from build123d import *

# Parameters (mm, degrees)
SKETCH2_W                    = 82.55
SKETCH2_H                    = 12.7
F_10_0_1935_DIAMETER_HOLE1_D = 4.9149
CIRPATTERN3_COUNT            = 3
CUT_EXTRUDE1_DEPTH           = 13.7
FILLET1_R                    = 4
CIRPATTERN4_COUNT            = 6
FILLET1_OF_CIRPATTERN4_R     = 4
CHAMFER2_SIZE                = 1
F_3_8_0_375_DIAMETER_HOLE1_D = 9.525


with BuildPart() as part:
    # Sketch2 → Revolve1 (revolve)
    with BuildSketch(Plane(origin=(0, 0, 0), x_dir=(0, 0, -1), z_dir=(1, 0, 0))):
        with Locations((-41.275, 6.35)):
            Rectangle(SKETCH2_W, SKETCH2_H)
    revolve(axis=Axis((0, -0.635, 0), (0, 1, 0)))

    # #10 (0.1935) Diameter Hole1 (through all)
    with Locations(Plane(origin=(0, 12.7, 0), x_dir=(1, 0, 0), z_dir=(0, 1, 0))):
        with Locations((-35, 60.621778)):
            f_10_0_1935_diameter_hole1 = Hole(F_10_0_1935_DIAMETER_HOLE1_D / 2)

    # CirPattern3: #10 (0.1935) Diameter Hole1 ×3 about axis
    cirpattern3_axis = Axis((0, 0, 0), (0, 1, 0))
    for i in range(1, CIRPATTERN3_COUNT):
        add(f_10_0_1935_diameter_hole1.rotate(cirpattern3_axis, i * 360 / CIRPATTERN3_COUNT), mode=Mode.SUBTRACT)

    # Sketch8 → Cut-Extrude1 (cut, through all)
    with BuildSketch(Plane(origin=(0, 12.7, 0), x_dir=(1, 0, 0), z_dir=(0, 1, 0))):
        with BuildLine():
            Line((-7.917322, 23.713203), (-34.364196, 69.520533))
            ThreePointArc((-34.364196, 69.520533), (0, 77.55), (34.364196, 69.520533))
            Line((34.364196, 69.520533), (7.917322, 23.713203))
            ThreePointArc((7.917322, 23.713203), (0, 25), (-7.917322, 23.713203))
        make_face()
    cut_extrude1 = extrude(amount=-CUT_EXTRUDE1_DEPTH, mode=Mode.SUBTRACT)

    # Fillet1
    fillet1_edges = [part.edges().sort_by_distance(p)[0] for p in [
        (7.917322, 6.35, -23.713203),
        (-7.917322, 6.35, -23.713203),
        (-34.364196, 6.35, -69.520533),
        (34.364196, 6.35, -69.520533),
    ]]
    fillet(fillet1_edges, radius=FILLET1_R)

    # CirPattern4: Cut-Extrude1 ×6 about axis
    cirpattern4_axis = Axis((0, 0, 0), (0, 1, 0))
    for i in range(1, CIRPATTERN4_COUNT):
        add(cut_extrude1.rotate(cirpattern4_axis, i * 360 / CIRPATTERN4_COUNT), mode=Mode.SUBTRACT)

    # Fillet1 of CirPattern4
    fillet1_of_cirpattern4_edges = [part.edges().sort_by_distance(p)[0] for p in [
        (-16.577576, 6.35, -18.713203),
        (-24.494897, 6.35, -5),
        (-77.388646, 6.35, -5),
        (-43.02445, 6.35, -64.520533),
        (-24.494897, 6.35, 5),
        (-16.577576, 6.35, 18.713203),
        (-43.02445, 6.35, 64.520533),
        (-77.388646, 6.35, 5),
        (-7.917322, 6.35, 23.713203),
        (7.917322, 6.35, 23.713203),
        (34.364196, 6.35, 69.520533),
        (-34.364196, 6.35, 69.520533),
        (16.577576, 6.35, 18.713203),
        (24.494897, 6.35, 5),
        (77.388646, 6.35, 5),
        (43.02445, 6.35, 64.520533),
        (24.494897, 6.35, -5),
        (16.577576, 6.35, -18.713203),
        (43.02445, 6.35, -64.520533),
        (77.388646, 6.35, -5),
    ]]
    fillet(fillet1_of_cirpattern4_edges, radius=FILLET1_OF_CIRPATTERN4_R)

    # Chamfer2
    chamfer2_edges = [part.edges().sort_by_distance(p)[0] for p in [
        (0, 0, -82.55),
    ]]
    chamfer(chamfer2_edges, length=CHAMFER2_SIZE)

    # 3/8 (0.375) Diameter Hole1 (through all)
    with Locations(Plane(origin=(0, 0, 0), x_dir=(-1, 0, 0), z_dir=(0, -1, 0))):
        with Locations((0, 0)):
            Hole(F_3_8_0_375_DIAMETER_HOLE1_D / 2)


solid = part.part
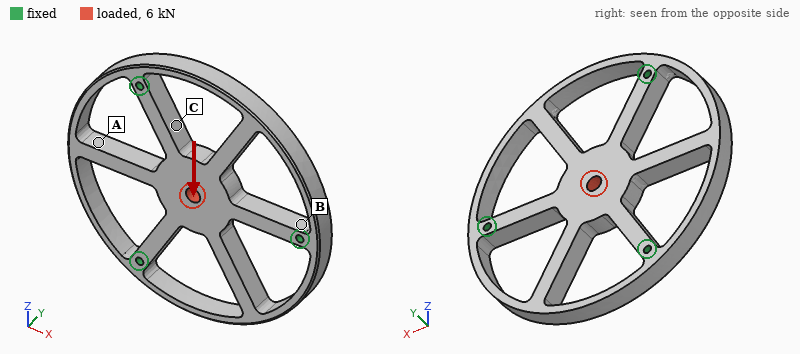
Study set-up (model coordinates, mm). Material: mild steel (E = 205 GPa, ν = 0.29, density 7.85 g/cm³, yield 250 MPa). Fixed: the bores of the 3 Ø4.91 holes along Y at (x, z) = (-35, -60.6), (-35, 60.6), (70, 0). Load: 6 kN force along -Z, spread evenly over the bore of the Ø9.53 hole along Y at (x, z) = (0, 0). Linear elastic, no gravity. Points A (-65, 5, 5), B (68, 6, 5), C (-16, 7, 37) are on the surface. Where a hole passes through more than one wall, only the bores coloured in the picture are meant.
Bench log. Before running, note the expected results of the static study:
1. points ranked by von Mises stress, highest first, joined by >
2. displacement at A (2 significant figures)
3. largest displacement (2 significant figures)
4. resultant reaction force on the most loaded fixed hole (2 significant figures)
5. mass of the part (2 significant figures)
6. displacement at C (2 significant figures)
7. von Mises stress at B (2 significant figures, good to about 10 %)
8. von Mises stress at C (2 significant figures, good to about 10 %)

C > B > A
4.0 µm
9.0 µm
3.2 kN
750 g
4.9 µm
14 MPa
24 MPa
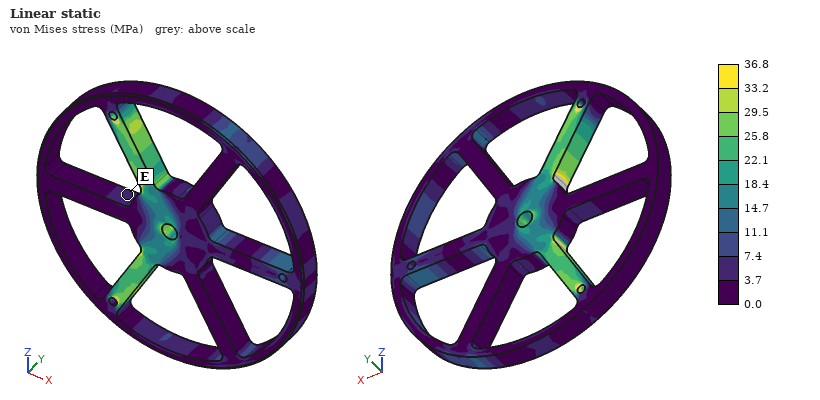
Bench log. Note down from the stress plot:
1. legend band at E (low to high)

3.7 to 7.4 MPa
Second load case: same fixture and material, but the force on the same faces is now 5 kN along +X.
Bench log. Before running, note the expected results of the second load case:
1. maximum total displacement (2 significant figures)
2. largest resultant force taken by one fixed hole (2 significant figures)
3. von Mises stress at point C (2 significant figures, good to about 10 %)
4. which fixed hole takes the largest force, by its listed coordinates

7.6 µm
3.1 kN
14 MPa
(70, 0)
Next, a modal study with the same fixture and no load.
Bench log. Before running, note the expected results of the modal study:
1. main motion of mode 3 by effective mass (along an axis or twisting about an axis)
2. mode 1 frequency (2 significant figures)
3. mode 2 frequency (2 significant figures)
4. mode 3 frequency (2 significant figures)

along Y
1800 Hz
1800 Hz
2000 Hz
